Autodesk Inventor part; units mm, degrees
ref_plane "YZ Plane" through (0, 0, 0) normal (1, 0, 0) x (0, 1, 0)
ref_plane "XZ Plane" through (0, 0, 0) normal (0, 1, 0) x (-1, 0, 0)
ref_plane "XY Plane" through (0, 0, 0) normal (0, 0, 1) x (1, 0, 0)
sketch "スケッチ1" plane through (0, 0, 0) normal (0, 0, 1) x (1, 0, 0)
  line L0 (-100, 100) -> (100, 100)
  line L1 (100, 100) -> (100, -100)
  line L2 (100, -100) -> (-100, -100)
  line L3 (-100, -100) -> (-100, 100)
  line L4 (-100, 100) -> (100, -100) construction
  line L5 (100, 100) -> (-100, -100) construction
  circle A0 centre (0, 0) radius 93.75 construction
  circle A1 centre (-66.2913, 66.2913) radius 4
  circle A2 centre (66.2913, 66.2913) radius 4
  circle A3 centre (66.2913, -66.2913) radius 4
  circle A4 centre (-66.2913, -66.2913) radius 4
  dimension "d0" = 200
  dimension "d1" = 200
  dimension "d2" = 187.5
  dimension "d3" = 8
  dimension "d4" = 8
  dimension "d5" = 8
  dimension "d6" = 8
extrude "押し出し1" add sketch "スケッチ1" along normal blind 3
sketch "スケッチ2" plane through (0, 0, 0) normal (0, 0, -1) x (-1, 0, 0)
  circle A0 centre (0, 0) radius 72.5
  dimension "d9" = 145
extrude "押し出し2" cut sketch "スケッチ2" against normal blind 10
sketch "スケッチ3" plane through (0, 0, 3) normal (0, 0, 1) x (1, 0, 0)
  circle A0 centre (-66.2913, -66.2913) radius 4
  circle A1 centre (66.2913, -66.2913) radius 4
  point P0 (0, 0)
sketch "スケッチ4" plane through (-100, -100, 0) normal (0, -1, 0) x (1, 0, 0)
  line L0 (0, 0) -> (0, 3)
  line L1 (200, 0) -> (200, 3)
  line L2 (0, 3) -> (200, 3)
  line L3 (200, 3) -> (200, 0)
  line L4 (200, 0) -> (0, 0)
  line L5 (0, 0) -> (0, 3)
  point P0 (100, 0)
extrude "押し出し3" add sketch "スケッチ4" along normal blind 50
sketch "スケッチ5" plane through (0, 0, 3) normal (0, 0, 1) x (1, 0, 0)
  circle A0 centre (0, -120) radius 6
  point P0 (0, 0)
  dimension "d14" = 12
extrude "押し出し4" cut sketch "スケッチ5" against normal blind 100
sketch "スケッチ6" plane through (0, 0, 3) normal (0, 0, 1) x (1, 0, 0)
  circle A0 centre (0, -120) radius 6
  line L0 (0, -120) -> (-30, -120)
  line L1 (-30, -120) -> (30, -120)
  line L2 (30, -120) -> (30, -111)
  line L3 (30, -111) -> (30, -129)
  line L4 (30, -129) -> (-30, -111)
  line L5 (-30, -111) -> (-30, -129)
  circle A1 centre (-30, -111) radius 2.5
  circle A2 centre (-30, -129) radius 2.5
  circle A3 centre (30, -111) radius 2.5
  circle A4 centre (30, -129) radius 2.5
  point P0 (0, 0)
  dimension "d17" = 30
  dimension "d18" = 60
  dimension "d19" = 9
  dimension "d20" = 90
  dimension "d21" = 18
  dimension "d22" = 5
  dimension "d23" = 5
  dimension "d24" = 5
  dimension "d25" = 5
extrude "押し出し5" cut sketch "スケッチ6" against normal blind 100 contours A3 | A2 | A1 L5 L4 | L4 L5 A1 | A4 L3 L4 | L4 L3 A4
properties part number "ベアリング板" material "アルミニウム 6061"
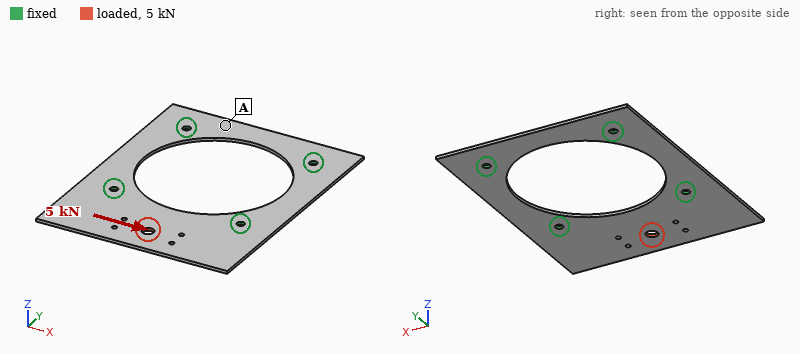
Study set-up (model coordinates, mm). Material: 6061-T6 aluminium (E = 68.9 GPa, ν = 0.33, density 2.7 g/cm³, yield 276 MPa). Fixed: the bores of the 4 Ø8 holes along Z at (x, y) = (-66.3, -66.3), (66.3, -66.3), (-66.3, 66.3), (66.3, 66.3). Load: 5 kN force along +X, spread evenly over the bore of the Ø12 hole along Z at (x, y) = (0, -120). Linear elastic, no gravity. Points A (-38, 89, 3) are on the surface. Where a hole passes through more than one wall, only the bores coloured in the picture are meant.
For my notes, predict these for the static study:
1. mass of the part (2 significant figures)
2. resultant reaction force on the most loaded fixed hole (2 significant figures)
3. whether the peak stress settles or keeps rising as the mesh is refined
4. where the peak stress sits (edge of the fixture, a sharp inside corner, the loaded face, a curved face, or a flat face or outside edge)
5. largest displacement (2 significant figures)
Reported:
270 g
3.0 kN
keeps rising
edge of the fixture
46 µm
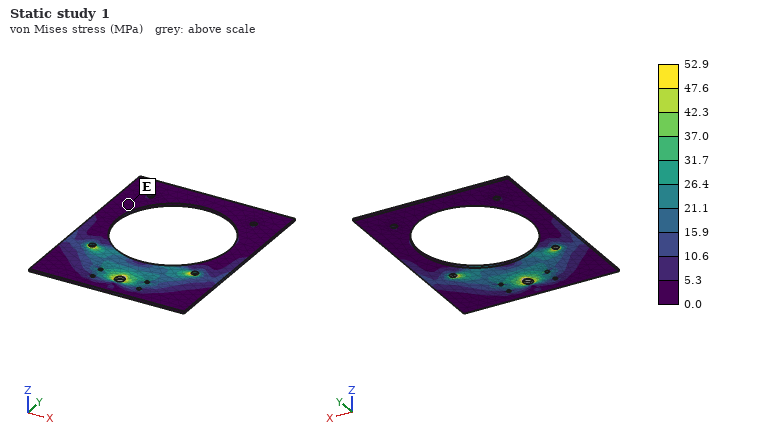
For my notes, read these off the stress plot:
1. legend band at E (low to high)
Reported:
0.0 to 5.3 MPa
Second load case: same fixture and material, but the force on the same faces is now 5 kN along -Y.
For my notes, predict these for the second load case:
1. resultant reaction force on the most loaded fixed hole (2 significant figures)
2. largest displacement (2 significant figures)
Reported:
3.0 kN
50 µm
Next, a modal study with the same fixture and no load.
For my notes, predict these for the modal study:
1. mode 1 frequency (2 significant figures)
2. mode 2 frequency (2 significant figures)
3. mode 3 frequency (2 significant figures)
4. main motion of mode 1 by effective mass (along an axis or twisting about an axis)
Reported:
290 Hz
470 Hz
680 Hz
along Z
